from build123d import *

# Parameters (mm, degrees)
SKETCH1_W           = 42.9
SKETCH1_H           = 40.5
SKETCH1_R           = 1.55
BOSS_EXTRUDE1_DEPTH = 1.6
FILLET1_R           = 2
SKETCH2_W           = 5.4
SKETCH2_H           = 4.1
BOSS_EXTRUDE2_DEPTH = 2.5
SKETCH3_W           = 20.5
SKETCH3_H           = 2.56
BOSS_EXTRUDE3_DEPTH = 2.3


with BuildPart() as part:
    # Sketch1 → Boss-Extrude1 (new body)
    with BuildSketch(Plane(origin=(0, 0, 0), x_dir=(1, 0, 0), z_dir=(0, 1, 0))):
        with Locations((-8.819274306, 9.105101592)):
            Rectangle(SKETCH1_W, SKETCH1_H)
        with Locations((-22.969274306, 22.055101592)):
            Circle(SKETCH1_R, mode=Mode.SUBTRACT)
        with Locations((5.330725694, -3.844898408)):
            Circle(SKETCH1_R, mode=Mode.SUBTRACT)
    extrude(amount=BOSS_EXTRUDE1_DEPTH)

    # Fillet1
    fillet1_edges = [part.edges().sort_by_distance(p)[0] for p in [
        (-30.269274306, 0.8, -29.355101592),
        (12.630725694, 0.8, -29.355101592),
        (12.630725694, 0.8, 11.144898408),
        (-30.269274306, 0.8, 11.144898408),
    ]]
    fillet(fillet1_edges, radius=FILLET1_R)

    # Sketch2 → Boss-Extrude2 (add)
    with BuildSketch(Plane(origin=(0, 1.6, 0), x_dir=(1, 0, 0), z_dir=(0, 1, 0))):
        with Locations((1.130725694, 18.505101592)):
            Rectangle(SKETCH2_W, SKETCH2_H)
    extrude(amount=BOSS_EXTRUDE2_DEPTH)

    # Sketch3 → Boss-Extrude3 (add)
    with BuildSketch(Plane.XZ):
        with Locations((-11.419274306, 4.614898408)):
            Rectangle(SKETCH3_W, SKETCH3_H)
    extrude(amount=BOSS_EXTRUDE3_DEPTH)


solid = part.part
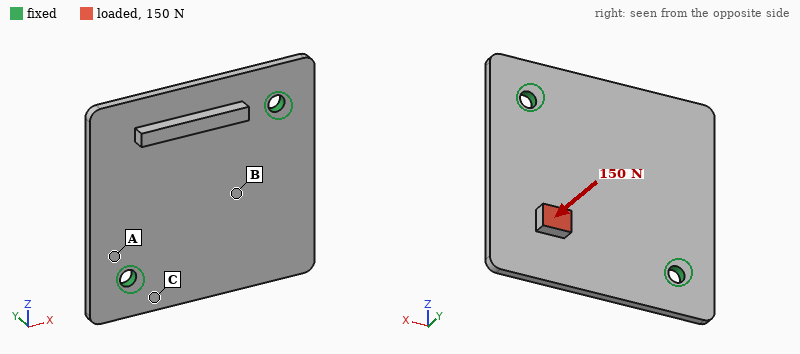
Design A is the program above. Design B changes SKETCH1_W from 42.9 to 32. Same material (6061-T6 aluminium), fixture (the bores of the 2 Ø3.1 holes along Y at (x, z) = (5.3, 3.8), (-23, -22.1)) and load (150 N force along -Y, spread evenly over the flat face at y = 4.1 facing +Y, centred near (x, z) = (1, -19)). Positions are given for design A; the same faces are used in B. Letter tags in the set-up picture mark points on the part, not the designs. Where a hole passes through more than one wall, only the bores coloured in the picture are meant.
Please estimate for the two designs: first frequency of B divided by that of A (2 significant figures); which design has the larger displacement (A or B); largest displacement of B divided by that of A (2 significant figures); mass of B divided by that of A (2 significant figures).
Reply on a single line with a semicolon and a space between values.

1.1; B; 1.1; 0.76
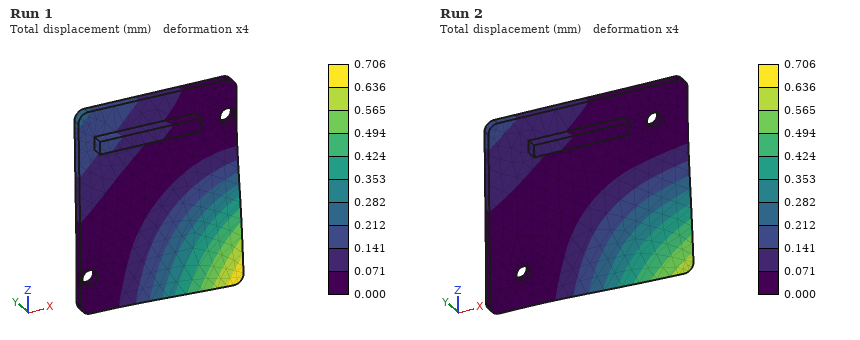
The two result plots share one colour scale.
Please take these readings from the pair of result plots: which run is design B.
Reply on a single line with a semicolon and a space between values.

Run 1
